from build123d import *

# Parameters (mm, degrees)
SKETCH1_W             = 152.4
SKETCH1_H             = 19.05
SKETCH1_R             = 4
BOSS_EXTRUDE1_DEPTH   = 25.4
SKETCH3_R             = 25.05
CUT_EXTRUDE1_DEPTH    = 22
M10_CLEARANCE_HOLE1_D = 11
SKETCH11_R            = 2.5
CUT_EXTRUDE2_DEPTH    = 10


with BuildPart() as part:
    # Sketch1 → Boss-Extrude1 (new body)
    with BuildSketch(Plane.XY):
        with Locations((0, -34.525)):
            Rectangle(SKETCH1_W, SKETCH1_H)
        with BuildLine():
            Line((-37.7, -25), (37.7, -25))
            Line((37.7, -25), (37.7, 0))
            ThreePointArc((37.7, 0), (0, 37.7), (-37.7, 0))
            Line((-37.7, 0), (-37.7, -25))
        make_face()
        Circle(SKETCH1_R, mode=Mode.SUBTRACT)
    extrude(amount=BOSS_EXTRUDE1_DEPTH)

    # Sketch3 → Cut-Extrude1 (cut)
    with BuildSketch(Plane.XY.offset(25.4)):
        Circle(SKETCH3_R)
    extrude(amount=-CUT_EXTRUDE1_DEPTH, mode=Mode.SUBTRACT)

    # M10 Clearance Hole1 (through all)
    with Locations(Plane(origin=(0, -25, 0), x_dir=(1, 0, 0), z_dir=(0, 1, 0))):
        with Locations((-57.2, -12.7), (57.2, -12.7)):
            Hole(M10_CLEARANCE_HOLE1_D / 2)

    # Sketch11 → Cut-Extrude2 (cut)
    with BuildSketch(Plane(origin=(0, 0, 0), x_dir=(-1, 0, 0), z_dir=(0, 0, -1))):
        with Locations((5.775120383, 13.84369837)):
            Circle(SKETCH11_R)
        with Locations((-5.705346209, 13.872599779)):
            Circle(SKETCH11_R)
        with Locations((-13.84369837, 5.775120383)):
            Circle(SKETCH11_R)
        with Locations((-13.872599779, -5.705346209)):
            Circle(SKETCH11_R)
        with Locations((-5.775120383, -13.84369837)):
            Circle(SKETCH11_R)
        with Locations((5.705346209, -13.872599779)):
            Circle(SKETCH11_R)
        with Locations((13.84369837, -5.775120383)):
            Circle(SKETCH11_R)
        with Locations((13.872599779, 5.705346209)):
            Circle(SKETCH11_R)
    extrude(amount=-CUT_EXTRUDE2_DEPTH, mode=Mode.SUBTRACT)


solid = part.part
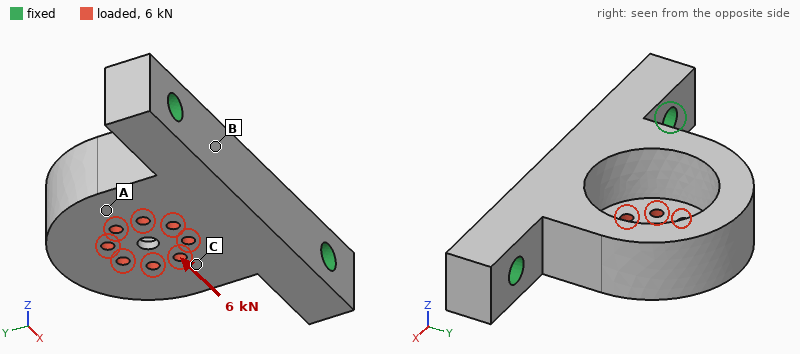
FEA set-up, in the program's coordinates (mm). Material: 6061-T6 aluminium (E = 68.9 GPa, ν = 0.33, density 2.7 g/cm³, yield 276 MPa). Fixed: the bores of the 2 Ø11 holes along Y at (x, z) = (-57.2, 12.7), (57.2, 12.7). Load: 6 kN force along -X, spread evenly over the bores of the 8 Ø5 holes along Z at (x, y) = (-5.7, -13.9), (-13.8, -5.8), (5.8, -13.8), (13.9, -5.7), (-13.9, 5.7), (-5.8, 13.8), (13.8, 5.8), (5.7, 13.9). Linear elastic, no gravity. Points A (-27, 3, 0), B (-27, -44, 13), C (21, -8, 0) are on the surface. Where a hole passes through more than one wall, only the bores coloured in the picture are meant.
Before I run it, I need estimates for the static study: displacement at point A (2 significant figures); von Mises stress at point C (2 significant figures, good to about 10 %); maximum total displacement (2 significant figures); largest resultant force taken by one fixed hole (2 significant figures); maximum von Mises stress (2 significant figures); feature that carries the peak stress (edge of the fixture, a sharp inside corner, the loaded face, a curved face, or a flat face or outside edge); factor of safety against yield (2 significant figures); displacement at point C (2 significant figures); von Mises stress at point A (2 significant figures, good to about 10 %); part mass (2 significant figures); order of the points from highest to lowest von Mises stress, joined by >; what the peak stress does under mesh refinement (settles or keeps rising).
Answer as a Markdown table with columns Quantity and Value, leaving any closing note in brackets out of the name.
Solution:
| Quantity | Value |
|---|---|
| displacement at point A | 24 µm |
| von Mises stress at point C | 27 MPa |
| maximum total displacement | 32 µm |
| largest resultant force taken by one fixed hole | 3.8 kN |
| maximum von Mises stress | 80 MPa |
| feature that carries the peak stress | the loaded face |
| factor of safety against yield | 3.4 |
| displacement at point C | 16 µm |
| von Mises stress at point A | 13 MPa |
| part mass | 350 g |
| order of the points from highest to lowest von Mises stress, joined by > | C > A > B |
| what the peak stress does under mesh refinement | settles |
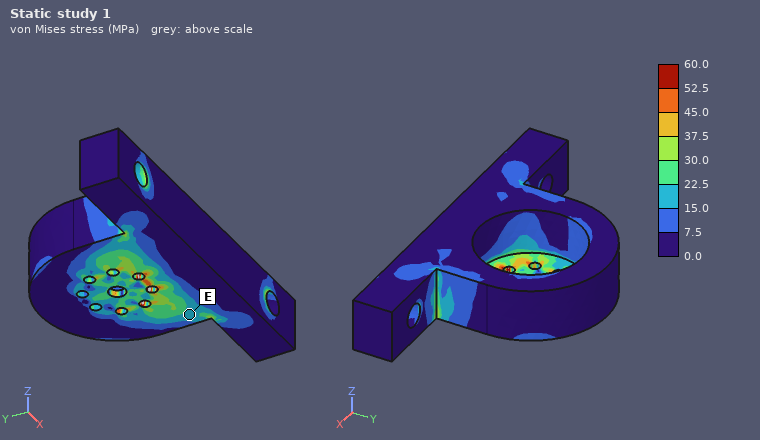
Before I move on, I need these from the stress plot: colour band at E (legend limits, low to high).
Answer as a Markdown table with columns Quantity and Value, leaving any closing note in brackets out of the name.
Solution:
| Quantity | Value |
|---|---|
| colour band at E | 15.0 to 22.5 MPa |
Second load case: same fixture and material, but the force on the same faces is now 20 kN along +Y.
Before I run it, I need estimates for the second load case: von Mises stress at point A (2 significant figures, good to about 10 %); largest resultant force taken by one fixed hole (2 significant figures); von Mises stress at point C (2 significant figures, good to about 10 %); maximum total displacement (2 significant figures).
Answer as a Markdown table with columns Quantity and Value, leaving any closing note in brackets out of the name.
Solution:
| Quantity | Value |
|---|---|
| von Mises stress at point A | 40 MPa |
| largest resultant force taken by one fixed hole | 11 kN |
| von Mises stress at point C | 74 MPa |
| maximum total displacement | 0.32 mm |
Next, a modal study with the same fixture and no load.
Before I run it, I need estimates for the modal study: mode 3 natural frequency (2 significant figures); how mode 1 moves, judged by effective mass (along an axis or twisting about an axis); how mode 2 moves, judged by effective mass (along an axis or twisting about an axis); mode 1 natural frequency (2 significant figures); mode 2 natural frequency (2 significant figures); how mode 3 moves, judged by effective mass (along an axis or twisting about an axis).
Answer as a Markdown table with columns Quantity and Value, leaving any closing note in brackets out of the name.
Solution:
| Quantity | Value |
|---|---|
| mode 3 natural frequency | 6300 Hz |
| how mode 1 moves, judged by effective mass | along Z |
| how mode 2 moves, judged by effective mass | along X |
| mode 1 natural frequency | 2000 Hz |
| mode 2 natural frequency | 5000 Hz |
| how mode 3 moves, judged by effective mass | along Y |
